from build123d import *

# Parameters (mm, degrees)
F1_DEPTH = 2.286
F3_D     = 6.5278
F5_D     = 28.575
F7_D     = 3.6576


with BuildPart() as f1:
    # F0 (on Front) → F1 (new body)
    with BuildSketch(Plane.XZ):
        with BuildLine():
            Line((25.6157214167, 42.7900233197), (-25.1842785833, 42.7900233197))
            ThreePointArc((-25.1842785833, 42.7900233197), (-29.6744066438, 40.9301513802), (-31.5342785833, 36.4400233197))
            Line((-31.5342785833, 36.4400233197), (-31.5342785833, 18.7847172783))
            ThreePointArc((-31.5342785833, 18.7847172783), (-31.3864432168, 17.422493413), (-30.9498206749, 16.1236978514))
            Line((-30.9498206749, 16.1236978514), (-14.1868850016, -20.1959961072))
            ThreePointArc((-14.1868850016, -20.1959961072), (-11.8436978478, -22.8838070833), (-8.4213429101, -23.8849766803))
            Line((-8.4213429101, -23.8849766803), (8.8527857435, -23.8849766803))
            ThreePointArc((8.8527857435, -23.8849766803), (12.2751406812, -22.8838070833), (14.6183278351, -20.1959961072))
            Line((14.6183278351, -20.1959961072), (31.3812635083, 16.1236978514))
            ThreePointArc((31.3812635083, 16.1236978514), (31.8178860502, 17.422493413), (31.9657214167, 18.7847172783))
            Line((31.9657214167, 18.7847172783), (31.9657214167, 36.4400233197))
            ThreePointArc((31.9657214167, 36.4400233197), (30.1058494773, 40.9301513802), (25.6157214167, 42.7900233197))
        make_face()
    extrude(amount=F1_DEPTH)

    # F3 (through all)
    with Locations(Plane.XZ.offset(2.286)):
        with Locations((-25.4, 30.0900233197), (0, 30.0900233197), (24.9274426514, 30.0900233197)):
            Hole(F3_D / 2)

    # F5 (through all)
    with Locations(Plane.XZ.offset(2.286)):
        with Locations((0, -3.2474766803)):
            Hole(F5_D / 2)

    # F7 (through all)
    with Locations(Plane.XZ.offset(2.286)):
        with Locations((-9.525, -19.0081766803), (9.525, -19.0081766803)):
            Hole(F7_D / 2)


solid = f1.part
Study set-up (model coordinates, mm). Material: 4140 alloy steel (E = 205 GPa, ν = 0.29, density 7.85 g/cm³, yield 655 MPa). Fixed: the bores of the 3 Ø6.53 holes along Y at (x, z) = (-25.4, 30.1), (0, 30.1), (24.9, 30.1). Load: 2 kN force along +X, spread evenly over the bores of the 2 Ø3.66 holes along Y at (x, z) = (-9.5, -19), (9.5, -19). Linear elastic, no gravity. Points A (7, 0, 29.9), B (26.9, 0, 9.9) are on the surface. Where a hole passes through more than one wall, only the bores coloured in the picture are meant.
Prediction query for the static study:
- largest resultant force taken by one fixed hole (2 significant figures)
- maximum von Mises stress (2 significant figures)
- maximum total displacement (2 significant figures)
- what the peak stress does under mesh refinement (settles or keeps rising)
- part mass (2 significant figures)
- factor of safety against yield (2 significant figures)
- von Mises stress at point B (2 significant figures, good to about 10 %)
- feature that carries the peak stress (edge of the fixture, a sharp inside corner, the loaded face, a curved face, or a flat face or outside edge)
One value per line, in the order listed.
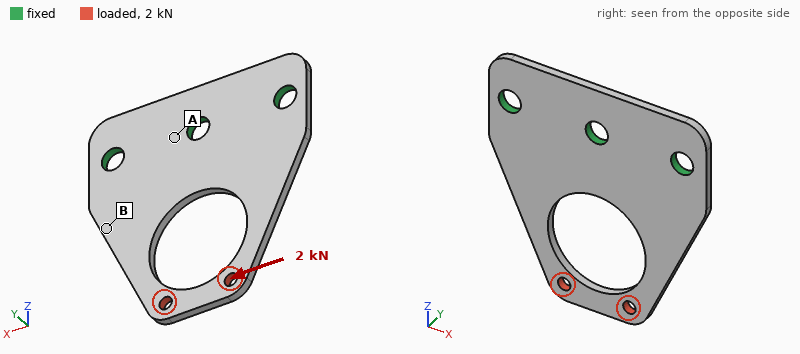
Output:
1.9 kN
430 MPa
81 µm
settles
48 g
1.5
110 MPa
a curved face
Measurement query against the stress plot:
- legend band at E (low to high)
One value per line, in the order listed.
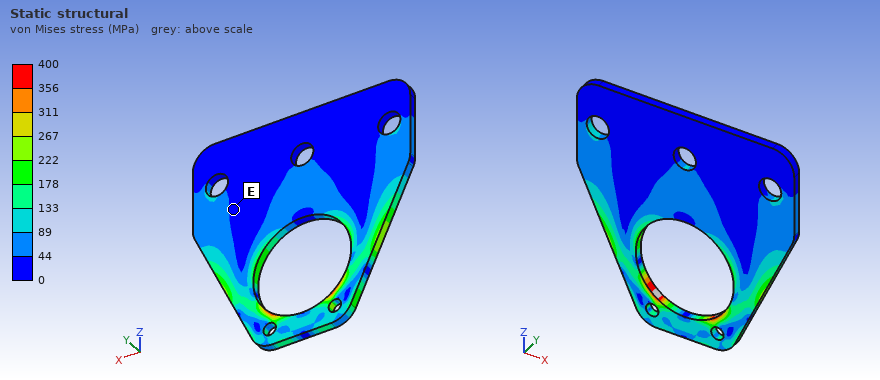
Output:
0 to 44 MPa
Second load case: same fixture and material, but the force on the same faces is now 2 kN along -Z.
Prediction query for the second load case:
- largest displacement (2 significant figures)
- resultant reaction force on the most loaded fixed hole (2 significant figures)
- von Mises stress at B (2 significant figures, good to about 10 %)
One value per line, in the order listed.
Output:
23 µm
980 N
43 MPa
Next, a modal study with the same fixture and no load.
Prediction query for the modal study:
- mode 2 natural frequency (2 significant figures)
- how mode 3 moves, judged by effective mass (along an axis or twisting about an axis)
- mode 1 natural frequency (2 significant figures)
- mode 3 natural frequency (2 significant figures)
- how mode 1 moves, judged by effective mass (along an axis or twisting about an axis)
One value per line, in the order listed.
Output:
2500 Hz
along Y
1000 Hz
4000 Hz
along Y
